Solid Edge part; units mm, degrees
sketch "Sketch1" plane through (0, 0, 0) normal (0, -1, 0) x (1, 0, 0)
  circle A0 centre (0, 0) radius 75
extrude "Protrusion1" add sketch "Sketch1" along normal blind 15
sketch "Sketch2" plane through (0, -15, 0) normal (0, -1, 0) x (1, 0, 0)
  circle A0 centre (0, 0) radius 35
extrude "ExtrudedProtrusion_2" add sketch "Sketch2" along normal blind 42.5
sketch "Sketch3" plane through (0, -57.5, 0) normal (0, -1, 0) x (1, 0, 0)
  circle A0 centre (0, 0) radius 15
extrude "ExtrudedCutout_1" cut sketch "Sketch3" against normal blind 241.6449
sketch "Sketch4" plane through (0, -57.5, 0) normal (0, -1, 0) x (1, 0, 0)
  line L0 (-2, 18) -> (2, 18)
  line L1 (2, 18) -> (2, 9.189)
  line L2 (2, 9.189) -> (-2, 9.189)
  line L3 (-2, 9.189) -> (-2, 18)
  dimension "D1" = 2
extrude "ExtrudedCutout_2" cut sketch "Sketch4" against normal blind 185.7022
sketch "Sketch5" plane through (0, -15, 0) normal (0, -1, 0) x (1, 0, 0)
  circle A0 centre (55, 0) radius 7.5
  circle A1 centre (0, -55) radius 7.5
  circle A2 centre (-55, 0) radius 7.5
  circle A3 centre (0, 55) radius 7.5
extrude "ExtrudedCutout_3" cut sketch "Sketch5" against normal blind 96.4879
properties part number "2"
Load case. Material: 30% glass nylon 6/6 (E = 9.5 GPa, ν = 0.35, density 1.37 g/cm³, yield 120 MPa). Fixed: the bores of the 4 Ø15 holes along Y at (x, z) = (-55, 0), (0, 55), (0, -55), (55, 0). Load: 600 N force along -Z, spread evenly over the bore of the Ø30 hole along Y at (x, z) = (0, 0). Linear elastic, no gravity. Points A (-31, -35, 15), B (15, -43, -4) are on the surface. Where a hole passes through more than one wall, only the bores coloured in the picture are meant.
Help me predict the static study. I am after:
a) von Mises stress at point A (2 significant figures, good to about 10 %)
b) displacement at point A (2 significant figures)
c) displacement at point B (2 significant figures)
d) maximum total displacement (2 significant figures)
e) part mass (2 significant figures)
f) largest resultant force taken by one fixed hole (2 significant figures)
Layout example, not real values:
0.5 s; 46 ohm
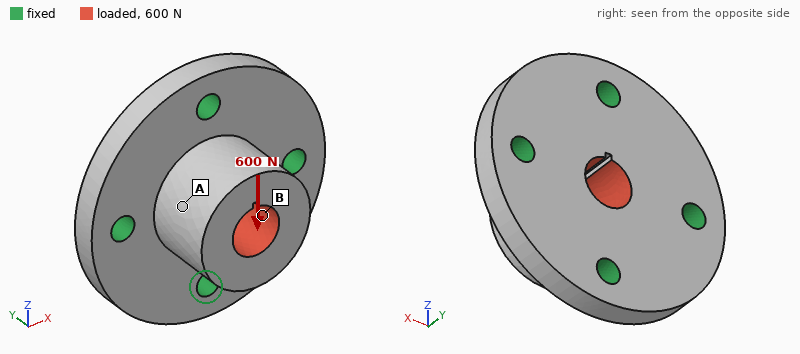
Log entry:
0.14 MPa; 3.3 µm; 4.1 µm; 5.9 µm; 520 g; 240 N
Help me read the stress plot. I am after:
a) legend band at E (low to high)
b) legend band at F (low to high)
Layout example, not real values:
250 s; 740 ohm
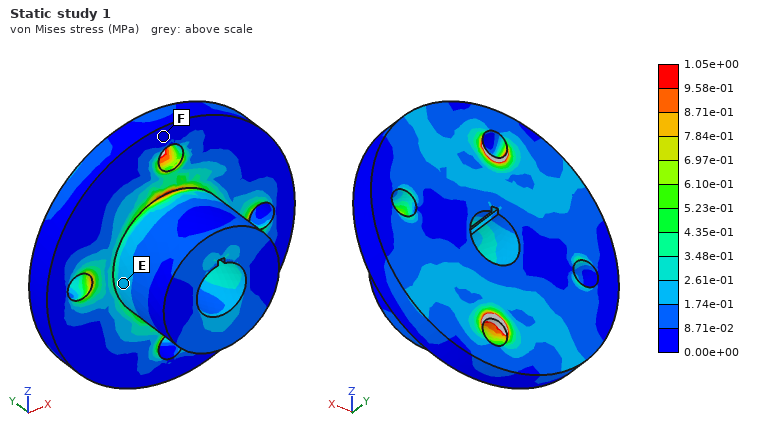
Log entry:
1.74e-01 to 2.61e-01 MPa; 0.00e+00 to 8.71e-02 MPa
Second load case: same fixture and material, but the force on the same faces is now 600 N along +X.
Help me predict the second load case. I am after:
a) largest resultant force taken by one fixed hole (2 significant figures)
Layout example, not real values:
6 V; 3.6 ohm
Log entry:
240 N
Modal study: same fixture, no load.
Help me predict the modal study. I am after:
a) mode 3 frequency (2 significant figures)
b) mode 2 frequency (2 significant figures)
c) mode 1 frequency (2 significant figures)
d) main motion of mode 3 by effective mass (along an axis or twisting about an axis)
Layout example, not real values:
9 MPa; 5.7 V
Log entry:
4000 Hz; 3600 Hz; 3600 Hz; along Y
